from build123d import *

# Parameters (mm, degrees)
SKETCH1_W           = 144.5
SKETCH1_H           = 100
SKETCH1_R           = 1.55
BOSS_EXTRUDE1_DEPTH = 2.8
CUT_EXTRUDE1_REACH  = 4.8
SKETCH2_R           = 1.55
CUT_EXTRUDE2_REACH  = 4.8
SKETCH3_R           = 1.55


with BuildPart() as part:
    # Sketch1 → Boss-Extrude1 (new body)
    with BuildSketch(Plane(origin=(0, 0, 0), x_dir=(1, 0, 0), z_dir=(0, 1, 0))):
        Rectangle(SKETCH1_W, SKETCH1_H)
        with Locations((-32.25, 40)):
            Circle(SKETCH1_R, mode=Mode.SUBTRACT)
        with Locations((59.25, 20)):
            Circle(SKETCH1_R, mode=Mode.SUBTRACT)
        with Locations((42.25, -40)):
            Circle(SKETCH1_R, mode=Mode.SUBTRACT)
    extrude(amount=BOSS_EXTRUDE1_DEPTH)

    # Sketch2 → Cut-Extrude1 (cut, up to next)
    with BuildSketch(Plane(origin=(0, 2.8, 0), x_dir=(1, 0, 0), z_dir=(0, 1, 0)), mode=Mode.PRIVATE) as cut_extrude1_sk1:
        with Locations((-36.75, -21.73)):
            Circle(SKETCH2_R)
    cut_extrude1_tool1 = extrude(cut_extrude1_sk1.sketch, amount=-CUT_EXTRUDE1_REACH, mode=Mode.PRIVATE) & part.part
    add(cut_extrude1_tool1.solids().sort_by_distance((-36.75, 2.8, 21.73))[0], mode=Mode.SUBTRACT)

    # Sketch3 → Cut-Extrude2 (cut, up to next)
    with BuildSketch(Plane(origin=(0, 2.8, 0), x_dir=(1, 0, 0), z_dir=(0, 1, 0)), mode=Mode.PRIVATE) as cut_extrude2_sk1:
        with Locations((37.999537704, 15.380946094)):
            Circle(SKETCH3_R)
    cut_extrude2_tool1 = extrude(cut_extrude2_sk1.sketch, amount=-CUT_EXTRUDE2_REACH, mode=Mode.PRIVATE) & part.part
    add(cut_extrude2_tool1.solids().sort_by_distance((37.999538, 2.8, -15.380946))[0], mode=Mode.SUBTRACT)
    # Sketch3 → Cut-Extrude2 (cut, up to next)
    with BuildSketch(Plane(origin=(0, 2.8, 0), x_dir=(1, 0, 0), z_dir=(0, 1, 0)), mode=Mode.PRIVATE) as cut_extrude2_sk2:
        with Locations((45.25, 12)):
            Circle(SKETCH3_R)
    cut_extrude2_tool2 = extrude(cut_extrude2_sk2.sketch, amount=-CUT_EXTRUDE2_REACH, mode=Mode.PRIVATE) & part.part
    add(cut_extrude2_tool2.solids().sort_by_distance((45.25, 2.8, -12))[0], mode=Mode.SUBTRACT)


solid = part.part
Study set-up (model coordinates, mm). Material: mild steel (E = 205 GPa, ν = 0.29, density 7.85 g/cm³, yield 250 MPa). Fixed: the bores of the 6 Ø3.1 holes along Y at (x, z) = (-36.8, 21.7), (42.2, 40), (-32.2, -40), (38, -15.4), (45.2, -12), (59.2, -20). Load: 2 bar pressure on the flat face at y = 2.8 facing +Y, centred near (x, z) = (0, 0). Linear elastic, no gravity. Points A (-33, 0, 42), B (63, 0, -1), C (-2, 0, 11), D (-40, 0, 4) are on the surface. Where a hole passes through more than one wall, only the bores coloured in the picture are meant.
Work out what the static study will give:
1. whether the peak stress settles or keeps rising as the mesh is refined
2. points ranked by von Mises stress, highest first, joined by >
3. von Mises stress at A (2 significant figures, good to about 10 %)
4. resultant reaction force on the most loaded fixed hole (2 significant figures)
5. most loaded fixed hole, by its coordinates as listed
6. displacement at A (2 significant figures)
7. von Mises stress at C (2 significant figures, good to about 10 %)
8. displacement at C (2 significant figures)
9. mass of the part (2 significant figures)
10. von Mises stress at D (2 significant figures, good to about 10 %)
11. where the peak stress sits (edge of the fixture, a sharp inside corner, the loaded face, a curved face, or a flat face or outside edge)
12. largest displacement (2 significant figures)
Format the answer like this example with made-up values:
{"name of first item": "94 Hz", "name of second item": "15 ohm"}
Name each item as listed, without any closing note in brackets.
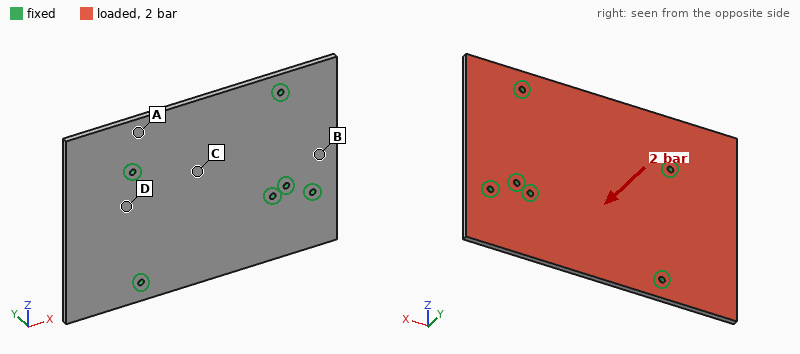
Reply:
{"whether the peak stress settles or keeps rising as the mesh is refined": "keeps rising", "points ranked by von Mises stress, highest first, joined by >": "D > A > C > B", "von Mises stress at A": "50 MPa", "resultant reaction force on the most loaded fixed hole": "920 N", "most loaded fixed hole, by its coordinates as listed": "(-36.8, 21.7)", "displacement at A": "0.031 mm", "von Mises stress at C": "30 MPa", "displacement at C": "0.052 mm", "mass of the part": "320 g", "von Mises stress at D": "62 MPa", "where the peak stress sits": "edge of the fixture", "largest displacement": "0.17 mm"}
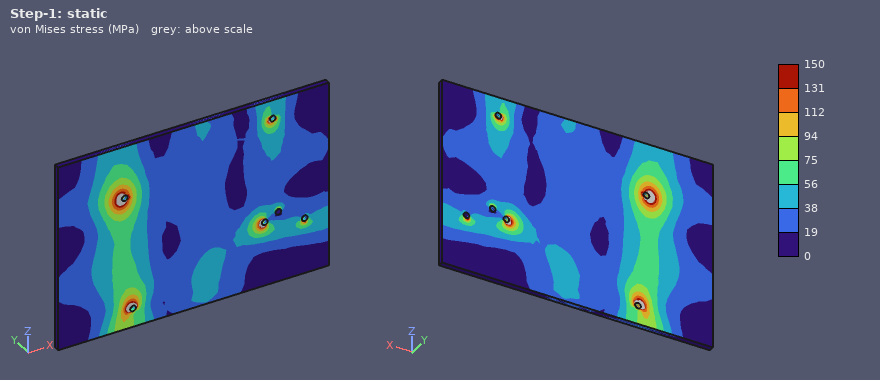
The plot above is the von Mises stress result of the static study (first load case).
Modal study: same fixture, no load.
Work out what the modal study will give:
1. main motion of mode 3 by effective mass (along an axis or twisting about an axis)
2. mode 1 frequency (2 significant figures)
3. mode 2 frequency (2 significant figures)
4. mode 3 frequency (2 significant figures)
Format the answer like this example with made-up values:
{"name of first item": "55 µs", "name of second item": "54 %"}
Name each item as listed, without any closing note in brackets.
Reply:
{"main motion of mode 3 by effective mass": "along Y", "mode 1 frequency": "1300 Hz", "mode 2 frequency": "1700 Hz", "mode 3 frequency": "2000 Hz"}
